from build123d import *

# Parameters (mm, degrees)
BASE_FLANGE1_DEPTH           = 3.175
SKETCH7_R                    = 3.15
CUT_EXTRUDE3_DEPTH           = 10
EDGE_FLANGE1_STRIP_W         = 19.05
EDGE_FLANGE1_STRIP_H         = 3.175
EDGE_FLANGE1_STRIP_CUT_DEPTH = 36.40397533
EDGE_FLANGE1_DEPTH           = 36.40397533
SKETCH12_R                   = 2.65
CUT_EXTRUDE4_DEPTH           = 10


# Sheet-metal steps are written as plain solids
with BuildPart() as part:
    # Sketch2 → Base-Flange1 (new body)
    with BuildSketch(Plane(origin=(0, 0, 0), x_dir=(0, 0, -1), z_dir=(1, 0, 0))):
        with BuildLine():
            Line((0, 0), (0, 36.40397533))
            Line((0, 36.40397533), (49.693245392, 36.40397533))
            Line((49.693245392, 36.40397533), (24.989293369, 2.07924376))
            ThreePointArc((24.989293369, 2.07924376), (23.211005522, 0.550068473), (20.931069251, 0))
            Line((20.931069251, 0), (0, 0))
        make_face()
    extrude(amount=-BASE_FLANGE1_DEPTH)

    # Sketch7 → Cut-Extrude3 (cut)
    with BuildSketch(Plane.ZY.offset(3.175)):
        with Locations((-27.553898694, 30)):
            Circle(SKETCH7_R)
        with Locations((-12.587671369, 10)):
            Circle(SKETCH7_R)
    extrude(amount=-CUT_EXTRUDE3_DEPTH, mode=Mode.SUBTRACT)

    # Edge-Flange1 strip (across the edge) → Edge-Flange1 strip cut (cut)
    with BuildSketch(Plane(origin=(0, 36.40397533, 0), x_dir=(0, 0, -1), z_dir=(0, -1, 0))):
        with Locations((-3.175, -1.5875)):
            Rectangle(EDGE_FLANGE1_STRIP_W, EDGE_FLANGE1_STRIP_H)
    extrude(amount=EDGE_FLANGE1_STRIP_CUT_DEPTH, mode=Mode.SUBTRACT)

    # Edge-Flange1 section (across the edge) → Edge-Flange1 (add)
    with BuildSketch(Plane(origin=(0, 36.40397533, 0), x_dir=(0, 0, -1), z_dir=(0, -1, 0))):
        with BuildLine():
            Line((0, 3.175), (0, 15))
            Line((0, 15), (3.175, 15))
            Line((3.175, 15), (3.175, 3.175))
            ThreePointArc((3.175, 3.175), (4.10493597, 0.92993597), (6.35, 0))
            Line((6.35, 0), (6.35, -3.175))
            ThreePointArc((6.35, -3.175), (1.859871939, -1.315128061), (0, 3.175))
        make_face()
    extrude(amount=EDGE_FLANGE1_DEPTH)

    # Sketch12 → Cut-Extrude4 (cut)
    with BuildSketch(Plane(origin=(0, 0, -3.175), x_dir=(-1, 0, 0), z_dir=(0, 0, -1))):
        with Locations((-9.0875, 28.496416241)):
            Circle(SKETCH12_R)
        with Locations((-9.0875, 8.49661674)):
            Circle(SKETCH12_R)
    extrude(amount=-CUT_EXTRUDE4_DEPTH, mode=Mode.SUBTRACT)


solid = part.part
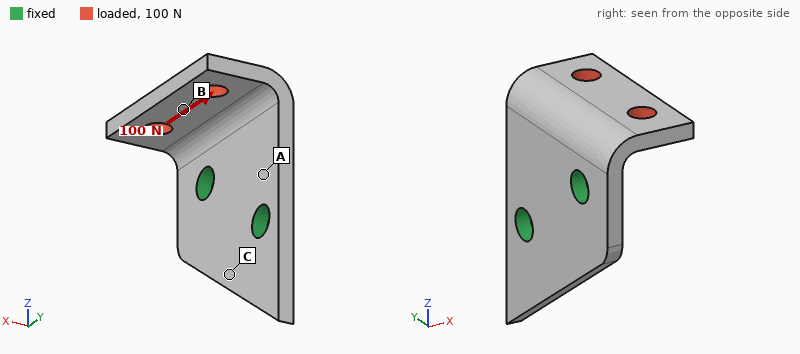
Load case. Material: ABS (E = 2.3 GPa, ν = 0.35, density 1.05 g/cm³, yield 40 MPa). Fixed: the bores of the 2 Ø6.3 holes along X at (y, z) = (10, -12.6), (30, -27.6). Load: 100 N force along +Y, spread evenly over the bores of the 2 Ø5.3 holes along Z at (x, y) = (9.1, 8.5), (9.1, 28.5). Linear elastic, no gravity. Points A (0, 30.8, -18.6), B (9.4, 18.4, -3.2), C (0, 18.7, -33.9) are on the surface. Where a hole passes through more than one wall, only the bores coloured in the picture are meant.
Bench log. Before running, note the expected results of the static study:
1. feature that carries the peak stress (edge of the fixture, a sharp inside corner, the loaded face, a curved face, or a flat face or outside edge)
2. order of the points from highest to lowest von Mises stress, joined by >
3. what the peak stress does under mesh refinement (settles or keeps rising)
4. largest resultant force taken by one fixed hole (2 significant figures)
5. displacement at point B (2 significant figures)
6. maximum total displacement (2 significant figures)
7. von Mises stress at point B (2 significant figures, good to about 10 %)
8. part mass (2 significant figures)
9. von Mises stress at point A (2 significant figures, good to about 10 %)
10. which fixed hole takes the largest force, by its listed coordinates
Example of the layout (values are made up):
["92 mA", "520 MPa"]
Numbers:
["edge of the fixture", "A > B > C", "keeps rising", "110 N", "0.32 mm", "0.77 mm", "3.9 MPa", "5.7 g", "6.6 MPa", "(10, -12.6)"]
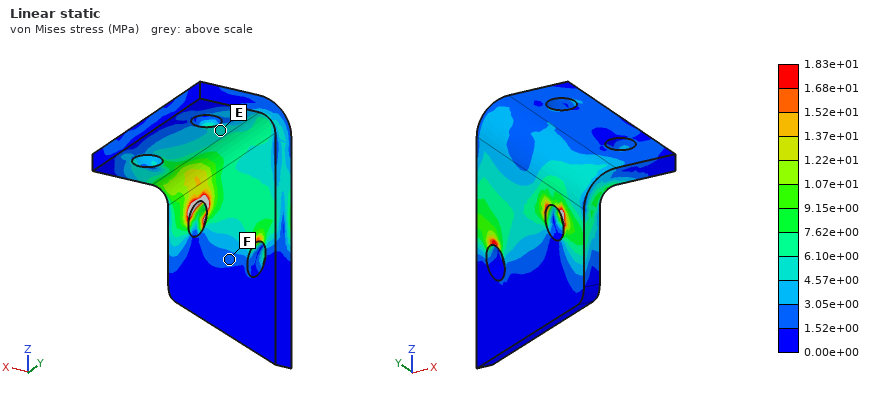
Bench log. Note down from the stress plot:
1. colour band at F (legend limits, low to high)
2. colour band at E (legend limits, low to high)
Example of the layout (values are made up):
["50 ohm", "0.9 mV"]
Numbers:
["1.52e+00 to 3.05e+00 MPa", "4.57e+00 to 6.10e+00 MPa"]
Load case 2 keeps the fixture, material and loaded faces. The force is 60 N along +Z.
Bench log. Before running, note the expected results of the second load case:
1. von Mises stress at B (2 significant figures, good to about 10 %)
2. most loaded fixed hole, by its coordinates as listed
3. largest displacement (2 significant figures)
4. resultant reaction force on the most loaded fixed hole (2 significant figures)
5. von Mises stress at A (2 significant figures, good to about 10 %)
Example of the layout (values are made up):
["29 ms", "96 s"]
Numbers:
["1.6 MPa", "(10, -12.6)", "0.74 mm", "36 N", "3.7 MPa"]
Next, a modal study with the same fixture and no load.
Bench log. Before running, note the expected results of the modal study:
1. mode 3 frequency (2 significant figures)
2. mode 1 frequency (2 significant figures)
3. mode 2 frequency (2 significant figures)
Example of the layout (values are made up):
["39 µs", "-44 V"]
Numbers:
["3100 Hz", "1200 Hz", "1900 Hz"]
